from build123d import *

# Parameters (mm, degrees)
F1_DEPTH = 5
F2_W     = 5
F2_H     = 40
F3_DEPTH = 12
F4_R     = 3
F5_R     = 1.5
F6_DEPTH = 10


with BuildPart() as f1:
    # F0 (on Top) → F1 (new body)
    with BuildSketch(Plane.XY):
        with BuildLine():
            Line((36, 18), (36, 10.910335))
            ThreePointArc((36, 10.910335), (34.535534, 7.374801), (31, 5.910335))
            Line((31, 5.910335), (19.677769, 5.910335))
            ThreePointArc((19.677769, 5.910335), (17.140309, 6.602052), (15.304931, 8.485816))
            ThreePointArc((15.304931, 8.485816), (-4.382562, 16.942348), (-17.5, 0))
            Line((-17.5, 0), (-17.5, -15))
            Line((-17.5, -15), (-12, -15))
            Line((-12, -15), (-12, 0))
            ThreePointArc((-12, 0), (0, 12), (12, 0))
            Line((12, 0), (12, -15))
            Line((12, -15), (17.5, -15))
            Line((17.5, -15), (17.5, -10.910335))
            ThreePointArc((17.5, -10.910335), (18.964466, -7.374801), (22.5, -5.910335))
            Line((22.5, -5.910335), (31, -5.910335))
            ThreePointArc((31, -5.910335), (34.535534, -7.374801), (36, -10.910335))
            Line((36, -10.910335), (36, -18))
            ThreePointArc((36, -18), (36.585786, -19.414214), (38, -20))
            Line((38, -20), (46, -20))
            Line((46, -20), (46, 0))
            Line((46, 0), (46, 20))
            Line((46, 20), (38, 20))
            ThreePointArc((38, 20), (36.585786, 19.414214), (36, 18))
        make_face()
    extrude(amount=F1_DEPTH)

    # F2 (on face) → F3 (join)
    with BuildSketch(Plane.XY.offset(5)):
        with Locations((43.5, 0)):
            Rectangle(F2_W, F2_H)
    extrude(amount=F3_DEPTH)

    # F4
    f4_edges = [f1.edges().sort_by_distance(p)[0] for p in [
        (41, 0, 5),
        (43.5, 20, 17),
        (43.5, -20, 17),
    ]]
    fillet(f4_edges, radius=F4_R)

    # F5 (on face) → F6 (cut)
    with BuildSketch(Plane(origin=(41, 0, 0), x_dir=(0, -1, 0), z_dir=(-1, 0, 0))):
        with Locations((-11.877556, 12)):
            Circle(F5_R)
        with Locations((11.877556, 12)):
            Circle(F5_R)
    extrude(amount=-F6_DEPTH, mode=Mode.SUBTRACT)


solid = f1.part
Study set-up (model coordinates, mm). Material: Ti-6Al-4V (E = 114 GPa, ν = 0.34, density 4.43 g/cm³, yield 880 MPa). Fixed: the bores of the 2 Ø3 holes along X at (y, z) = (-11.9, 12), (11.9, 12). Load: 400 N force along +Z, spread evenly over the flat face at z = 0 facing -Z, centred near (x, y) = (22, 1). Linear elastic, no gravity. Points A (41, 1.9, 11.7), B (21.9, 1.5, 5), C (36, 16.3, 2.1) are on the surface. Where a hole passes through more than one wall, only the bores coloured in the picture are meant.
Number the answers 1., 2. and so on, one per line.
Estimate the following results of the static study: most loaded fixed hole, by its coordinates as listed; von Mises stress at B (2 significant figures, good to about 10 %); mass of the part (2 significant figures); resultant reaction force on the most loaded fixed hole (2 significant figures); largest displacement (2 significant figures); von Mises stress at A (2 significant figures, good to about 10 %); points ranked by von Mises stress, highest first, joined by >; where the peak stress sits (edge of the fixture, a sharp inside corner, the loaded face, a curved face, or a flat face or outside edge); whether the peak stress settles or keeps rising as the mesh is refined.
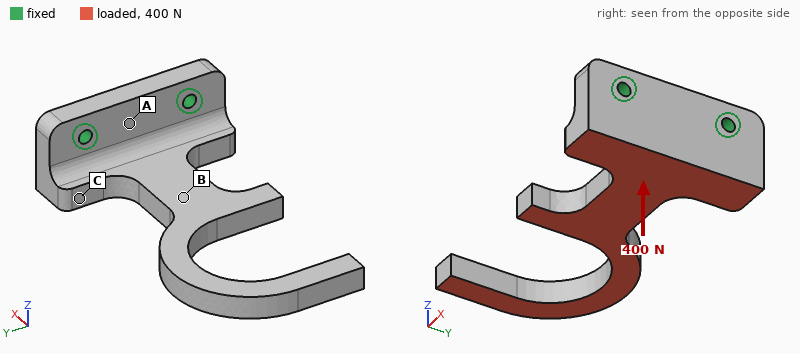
1. (11.9, 12)
2. 74 MPa
3. 34 g
4. 240 N
5. 0.81 mm
6. 23 MPa
7. B > A > C
8. edge of the fixture
9. keeps rising
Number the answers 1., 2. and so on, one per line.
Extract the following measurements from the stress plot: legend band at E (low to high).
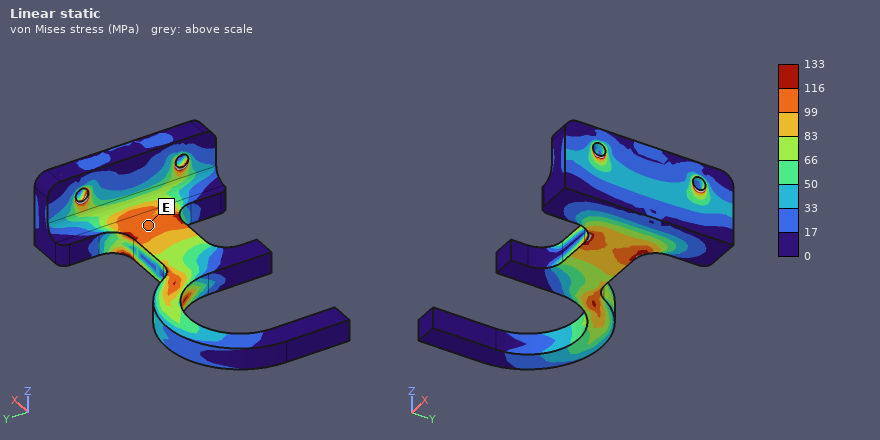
1. 99 to 116 MPa
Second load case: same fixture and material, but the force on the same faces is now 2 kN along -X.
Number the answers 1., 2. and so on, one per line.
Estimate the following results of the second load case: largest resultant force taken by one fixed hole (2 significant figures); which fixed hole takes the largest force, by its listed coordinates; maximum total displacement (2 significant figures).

1. 1.1 kN
2. (11.9, 12)
3. 0.80 mm
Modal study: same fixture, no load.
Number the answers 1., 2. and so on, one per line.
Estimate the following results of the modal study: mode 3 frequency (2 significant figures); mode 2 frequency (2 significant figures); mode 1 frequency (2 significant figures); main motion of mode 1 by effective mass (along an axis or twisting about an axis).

1. 2500 Hz
2. 1500 Hz
3. 910 Hz
4. along Z
